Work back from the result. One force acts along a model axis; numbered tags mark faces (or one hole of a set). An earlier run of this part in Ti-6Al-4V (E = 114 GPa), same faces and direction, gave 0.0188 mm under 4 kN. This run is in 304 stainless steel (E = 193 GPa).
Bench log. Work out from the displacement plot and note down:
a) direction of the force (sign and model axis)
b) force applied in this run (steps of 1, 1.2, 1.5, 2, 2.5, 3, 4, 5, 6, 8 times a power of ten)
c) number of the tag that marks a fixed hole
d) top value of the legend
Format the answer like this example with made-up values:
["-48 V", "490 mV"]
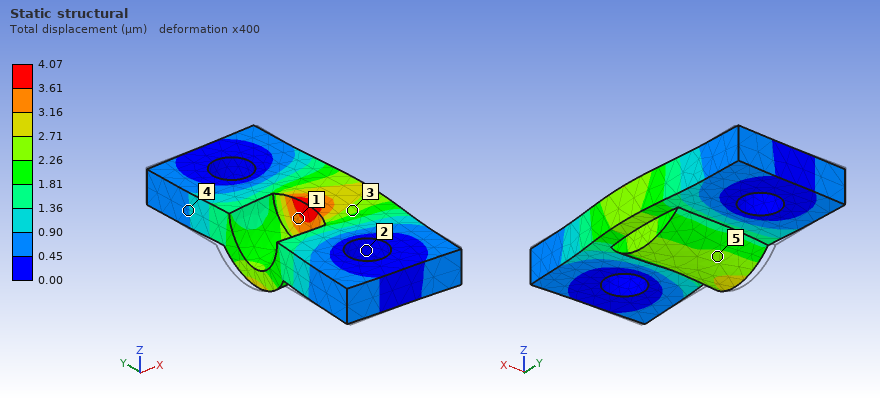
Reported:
["+X", "1.5 kN", "2", "4.07 µm"]
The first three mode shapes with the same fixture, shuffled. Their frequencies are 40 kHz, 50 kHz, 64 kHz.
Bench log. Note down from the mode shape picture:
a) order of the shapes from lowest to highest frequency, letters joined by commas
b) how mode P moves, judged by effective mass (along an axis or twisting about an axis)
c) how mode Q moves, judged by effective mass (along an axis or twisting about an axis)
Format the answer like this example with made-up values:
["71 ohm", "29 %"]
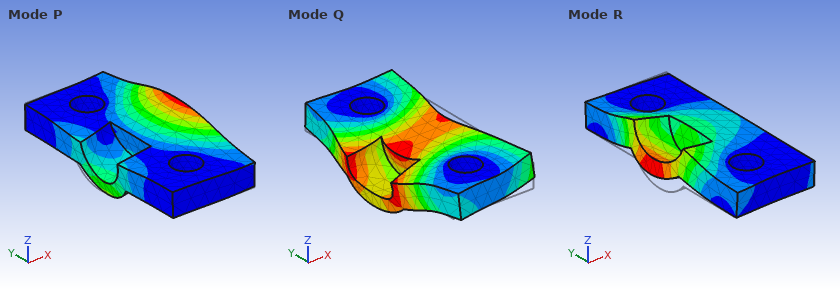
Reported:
["P, R, Q", "along Z", "along X"]
